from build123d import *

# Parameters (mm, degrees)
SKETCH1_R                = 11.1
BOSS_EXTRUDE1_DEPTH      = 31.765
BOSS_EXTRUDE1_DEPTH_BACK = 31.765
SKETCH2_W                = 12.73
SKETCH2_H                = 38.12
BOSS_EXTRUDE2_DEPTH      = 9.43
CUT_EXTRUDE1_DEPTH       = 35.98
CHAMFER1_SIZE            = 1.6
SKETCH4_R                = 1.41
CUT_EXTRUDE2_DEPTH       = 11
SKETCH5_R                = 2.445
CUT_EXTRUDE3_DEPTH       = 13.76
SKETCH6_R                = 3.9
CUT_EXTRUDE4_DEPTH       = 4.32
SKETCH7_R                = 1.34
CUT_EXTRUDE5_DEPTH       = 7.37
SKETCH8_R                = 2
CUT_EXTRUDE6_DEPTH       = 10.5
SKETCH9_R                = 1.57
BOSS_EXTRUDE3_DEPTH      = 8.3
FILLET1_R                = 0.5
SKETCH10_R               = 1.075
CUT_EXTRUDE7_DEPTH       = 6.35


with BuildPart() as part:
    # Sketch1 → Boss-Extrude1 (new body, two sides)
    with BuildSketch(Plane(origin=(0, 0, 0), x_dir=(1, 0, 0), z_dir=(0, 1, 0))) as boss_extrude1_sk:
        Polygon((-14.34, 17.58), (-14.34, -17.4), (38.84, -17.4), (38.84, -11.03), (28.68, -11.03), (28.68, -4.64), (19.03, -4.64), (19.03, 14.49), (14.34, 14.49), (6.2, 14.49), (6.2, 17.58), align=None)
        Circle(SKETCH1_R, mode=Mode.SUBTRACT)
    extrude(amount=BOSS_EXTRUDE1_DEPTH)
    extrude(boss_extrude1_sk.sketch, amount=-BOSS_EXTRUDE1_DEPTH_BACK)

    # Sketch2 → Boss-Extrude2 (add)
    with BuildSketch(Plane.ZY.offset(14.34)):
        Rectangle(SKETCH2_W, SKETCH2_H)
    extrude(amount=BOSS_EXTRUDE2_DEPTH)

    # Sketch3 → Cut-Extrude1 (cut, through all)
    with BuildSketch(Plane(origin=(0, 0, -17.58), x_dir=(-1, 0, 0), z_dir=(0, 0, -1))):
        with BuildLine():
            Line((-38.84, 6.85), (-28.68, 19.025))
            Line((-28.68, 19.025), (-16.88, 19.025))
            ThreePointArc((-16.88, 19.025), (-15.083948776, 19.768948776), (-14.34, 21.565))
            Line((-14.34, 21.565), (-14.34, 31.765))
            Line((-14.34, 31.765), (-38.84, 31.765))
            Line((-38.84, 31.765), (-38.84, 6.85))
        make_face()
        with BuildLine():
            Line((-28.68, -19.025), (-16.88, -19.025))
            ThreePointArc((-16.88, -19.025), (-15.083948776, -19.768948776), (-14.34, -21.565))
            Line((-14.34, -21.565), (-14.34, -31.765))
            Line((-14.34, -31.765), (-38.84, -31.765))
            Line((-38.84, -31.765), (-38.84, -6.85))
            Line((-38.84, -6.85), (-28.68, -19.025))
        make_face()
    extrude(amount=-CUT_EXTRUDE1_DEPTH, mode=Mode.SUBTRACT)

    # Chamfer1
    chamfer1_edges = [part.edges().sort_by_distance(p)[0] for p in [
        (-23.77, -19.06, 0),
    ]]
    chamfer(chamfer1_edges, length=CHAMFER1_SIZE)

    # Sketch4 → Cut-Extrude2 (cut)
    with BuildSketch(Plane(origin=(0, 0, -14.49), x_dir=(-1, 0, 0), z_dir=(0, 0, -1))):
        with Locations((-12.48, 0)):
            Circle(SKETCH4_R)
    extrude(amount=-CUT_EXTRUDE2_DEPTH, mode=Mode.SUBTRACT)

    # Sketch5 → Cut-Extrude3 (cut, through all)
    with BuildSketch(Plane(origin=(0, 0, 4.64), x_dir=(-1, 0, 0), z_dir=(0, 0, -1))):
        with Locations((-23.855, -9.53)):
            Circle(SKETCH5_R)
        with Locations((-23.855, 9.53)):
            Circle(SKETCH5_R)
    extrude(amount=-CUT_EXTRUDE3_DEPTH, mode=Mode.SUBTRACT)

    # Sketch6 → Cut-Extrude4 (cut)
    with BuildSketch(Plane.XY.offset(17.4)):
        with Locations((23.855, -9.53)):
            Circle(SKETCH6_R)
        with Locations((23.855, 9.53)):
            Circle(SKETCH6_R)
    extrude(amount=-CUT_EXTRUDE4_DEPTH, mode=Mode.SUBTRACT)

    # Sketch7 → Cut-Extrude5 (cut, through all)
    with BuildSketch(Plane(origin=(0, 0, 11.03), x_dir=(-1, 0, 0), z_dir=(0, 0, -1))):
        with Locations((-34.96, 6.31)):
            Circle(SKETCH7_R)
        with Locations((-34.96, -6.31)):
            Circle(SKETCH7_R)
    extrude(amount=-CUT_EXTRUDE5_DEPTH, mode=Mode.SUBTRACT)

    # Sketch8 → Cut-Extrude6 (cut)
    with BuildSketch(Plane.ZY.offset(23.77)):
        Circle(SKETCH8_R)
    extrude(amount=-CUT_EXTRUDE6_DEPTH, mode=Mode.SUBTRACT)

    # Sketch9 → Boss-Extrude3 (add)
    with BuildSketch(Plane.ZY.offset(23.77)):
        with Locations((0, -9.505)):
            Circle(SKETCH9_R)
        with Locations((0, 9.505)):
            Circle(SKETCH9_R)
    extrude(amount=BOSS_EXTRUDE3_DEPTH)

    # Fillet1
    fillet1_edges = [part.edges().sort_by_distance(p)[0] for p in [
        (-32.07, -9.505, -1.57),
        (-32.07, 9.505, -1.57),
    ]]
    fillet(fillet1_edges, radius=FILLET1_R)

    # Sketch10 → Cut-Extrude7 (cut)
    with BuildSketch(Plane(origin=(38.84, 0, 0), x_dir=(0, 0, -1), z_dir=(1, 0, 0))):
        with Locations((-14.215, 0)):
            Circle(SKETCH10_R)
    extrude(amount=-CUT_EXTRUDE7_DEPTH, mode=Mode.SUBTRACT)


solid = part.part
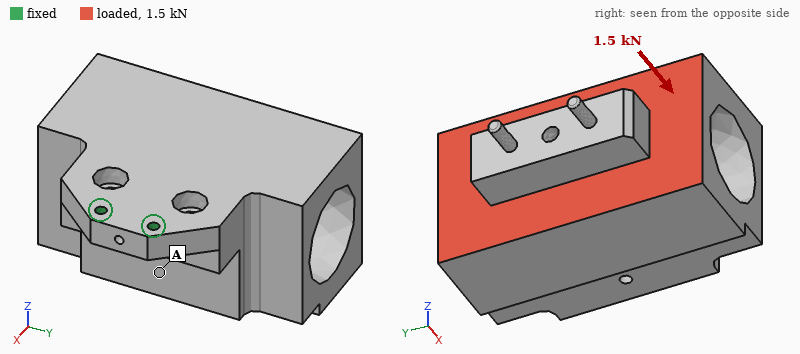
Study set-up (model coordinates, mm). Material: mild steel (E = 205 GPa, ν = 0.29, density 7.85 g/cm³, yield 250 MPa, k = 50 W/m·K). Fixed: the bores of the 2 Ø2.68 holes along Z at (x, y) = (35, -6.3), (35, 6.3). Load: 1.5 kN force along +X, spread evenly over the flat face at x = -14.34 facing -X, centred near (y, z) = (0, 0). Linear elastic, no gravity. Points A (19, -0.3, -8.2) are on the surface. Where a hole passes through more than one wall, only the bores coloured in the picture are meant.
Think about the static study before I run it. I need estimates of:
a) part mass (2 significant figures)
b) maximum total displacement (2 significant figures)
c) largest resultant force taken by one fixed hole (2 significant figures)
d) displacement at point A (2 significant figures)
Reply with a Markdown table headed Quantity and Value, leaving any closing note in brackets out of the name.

| Quantity | Value |
|---|---|
| part mass | 420 g |
| maximum total displacement | 0.14 mm |
| largest resultant force taken by one fixed hole | 750 N |
| displacement at point A | 0.056 mm |
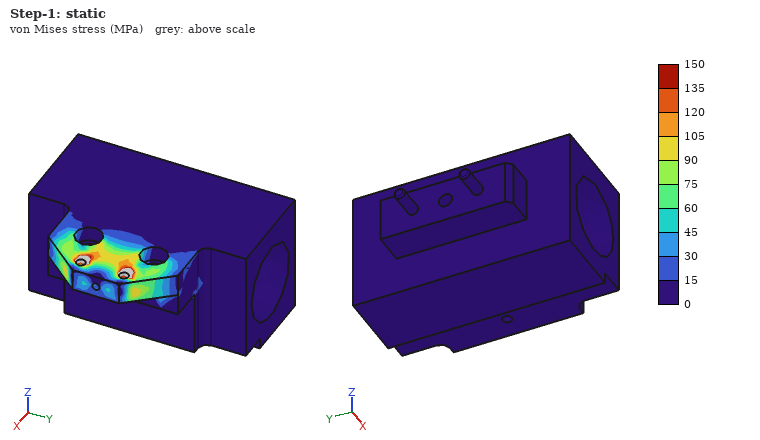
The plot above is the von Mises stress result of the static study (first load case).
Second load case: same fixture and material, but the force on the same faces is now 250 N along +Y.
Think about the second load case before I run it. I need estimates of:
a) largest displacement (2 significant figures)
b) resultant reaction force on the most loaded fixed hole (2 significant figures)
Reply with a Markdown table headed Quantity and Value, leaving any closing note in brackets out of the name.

| Quantity | Value |
|---|---|
| largest displacement | 10.0 µm |
| resultant reaction force on the most loaded fixed hole | 870 N |
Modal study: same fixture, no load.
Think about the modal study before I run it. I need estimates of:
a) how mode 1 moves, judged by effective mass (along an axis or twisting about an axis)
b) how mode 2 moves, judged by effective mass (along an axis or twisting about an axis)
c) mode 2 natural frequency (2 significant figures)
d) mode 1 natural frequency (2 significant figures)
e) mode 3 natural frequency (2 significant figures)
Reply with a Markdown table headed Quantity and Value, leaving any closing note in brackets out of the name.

| Quantity | Value |
|---|---|
| how mode 1 moves, judged by effective mass | along Z |
| how mode 2 moves, judged by effective mass | along Y |
| mode 2 natural frequency | 1700 Hz |
| mode 1 natural frequency | 680 Hz |
| mode 3 natural frequency | 2300 Hz |
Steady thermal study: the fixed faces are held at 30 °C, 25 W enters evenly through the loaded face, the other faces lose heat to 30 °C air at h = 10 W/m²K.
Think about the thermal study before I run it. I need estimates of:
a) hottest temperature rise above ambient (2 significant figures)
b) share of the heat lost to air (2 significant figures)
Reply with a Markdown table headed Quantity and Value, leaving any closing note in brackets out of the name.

| Quantity | Value |
|---|---|
| hottest temperature rise above ambient | 53 K |
| share of the heat lost to air | 25 % |
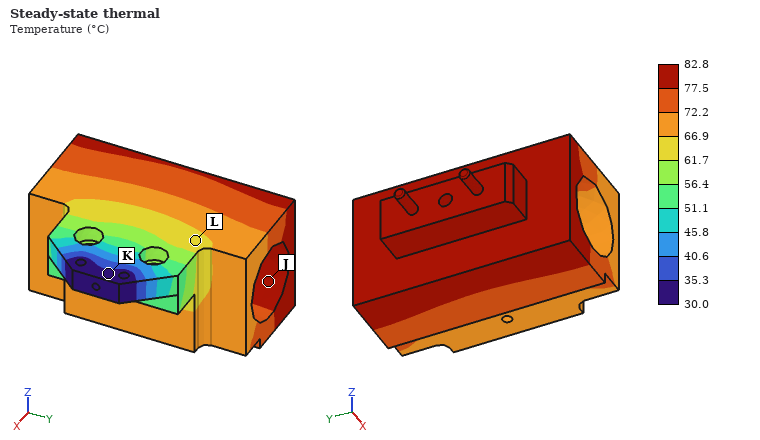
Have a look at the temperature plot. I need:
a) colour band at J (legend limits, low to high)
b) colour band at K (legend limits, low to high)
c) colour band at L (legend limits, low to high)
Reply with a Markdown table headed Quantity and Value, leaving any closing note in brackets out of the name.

| Quantity | Value |
|---|---|
| colour band at J | 77.5 to 82.8 °C |
| colour band at K | 30.0 to 35.3 °C |
| colour band at L | 61.7 to 66.9 °C |
